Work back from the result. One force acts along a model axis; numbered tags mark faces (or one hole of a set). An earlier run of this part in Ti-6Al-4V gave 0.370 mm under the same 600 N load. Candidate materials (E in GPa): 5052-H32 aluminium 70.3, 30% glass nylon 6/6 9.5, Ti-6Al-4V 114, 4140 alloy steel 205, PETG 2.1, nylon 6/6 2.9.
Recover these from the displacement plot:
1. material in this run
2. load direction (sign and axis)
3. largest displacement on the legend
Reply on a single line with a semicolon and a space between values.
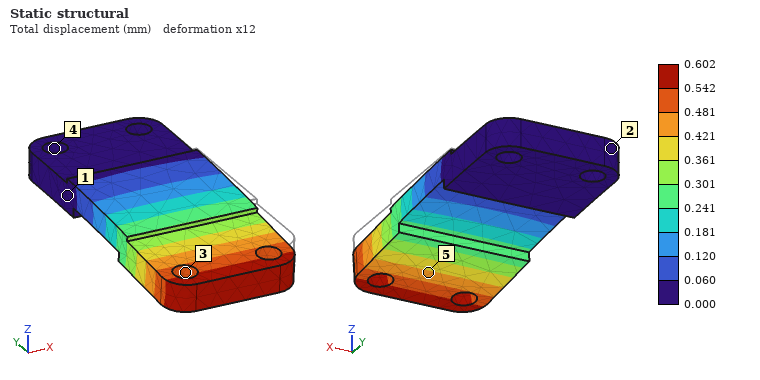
5052-H32 aluminium; -Z; 0.602 mm
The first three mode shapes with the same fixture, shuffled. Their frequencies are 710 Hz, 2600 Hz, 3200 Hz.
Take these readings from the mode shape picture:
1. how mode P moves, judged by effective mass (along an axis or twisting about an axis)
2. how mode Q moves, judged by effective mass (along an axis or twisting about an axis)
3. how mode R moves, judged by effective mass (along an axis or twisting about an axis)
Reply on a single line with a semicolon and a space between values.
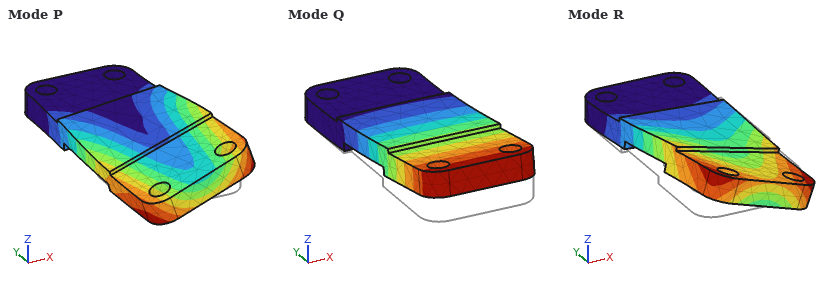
along X; along Z; along X
